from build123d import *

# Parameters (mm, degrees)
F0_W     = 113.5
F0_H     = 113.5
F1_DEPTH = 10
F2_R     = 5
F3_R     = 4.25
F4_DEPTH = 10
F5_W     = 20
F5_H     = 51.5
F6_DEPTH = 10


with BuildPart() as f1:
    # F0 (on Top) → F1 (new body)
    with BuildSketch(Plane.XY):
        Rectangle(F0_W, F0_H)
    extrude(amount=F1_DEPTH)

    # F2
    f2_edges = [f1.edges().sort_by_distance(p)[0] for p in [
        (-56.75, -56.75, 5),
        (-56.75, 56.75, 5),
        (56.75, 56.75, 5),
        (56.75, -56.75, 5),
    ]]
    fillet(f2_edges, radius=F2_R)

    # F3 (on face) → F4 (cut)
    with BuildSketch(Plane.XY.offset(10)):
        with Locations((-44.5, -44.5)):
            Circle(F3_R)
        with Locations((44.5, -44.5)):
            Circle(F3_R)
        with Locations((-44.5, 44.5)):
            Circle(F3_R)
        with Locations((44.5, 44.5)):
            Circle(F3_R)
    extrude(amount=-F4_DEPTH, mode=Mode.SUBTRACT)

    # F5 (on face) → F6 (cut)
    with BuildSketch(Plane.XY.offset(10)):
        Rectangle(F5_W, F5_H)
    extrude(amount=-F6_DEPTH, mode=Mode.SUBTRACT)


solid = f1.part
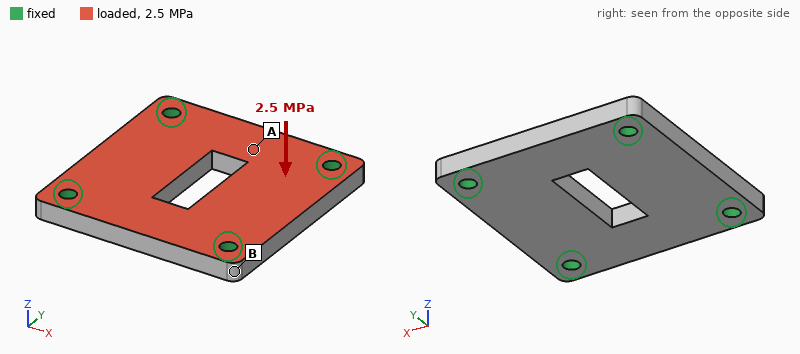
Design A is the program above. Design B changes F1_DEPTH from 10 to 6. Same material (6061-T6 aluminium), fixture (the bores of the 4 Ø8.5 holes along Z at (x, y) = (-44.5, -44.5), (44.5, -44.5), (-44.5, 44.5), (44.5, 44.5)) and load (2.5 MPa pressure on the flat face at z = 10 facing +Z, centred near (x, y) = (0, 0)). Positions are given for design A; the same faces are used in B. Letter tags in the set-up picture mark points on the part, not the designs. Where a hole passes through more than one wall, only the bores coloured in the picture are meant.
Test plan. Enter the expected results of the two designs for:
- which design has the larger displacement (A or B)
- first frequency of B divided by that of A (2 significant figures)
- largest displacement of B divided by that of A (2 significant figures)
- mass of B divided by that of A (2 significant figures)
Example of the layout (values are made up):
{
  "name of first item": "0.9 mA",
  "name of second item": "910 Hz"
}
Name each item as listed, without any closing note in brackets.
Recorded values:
{
  "which design has the larger displacement": "B",
  "first frequency of B divided by that of A": "0.65",
  "largest displacement of B divided by that of A": "4.0",
  "mass of B divided by that of A": "0.60"
}
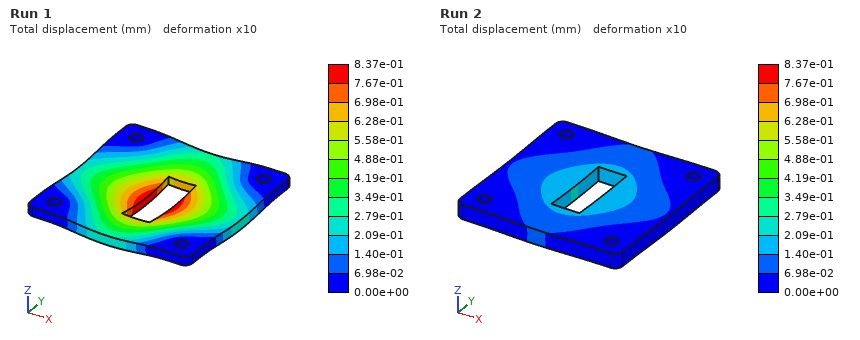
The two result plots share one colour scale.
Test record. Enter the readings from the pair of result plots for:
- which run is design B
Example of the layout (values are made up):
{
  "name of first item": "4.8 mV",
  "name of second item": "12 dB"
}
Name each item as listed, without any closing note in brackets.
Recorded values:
{
  "which run is design B": "Run 1"
}
